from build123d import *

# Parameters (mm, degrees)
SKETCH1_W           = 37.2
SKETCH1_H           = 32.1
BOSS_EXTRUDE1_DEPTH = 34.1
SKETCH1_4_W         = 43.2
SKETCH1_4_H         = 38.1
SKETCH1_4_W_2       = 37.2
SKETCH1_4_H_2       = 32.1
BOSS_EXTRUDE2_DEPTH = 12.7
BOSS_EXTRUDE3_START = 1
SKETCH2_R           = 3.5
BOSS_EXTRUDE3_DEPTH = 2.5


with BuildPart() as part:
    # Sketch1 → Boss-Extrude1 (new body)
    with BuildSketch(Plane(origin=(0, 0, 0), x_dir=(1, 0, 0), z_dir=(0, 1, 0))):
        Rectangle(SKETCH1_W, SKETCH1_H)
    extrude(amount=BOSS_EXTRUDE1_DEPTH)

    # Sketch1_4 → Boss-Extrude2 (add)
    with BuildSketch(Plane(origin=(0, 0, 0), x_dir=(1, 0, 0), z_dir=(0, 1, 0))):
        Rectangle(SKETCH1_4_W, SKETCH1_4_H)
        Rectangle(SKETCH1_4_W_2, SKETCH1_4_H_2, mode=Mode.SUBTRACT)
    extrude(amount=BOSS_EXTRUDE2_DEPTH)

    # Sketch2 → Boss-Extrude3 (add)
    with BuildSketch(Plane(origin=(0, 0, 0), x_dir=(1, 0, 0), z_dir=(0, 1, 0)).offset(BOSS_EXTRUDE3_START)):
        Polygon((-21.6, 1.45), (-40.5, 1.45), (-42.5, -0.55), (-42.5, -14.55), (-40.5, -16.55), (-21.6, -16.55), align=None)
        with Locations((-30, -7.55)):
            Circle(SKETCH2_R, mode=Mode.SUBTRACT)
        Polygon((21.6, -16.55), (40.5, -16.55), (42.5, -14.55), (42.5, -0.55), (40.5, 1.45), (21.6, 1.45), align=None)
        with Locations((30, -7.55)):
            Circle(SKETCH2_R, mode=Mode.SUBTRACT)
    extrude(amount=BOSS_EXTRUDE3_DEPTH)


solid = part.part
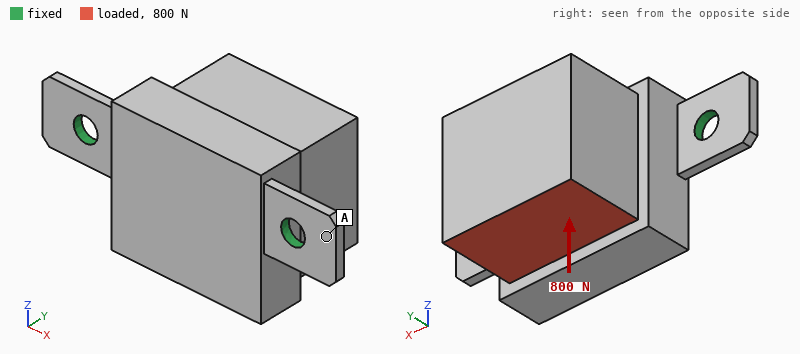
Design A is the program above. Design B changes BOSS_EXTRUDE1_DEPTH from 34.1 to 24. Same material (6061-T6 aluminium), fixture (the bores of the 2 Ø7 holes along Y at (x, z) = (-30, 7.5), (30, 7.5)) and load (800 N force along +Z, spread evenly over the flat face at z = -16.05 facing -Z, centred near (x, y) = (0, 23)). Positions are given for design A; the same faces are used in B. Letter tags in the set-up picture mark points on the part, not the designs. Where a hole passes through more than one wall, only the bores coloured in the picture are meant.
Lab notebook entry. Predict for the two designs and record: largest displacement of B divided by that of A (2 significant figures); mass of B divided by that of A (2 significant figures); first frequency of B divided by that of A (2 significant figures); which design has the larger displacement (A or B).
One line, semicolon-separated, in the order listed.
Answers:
0.62; 0.75; 1.4; A
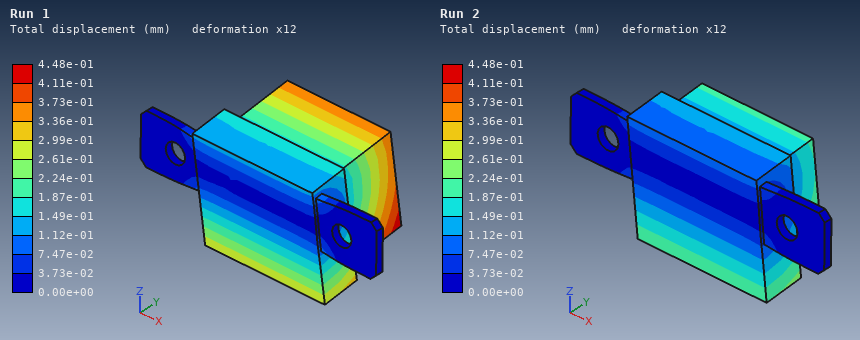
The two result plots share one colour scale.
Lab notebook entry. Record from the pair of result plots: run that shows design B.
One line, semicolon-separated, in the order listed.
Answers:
Run 2
